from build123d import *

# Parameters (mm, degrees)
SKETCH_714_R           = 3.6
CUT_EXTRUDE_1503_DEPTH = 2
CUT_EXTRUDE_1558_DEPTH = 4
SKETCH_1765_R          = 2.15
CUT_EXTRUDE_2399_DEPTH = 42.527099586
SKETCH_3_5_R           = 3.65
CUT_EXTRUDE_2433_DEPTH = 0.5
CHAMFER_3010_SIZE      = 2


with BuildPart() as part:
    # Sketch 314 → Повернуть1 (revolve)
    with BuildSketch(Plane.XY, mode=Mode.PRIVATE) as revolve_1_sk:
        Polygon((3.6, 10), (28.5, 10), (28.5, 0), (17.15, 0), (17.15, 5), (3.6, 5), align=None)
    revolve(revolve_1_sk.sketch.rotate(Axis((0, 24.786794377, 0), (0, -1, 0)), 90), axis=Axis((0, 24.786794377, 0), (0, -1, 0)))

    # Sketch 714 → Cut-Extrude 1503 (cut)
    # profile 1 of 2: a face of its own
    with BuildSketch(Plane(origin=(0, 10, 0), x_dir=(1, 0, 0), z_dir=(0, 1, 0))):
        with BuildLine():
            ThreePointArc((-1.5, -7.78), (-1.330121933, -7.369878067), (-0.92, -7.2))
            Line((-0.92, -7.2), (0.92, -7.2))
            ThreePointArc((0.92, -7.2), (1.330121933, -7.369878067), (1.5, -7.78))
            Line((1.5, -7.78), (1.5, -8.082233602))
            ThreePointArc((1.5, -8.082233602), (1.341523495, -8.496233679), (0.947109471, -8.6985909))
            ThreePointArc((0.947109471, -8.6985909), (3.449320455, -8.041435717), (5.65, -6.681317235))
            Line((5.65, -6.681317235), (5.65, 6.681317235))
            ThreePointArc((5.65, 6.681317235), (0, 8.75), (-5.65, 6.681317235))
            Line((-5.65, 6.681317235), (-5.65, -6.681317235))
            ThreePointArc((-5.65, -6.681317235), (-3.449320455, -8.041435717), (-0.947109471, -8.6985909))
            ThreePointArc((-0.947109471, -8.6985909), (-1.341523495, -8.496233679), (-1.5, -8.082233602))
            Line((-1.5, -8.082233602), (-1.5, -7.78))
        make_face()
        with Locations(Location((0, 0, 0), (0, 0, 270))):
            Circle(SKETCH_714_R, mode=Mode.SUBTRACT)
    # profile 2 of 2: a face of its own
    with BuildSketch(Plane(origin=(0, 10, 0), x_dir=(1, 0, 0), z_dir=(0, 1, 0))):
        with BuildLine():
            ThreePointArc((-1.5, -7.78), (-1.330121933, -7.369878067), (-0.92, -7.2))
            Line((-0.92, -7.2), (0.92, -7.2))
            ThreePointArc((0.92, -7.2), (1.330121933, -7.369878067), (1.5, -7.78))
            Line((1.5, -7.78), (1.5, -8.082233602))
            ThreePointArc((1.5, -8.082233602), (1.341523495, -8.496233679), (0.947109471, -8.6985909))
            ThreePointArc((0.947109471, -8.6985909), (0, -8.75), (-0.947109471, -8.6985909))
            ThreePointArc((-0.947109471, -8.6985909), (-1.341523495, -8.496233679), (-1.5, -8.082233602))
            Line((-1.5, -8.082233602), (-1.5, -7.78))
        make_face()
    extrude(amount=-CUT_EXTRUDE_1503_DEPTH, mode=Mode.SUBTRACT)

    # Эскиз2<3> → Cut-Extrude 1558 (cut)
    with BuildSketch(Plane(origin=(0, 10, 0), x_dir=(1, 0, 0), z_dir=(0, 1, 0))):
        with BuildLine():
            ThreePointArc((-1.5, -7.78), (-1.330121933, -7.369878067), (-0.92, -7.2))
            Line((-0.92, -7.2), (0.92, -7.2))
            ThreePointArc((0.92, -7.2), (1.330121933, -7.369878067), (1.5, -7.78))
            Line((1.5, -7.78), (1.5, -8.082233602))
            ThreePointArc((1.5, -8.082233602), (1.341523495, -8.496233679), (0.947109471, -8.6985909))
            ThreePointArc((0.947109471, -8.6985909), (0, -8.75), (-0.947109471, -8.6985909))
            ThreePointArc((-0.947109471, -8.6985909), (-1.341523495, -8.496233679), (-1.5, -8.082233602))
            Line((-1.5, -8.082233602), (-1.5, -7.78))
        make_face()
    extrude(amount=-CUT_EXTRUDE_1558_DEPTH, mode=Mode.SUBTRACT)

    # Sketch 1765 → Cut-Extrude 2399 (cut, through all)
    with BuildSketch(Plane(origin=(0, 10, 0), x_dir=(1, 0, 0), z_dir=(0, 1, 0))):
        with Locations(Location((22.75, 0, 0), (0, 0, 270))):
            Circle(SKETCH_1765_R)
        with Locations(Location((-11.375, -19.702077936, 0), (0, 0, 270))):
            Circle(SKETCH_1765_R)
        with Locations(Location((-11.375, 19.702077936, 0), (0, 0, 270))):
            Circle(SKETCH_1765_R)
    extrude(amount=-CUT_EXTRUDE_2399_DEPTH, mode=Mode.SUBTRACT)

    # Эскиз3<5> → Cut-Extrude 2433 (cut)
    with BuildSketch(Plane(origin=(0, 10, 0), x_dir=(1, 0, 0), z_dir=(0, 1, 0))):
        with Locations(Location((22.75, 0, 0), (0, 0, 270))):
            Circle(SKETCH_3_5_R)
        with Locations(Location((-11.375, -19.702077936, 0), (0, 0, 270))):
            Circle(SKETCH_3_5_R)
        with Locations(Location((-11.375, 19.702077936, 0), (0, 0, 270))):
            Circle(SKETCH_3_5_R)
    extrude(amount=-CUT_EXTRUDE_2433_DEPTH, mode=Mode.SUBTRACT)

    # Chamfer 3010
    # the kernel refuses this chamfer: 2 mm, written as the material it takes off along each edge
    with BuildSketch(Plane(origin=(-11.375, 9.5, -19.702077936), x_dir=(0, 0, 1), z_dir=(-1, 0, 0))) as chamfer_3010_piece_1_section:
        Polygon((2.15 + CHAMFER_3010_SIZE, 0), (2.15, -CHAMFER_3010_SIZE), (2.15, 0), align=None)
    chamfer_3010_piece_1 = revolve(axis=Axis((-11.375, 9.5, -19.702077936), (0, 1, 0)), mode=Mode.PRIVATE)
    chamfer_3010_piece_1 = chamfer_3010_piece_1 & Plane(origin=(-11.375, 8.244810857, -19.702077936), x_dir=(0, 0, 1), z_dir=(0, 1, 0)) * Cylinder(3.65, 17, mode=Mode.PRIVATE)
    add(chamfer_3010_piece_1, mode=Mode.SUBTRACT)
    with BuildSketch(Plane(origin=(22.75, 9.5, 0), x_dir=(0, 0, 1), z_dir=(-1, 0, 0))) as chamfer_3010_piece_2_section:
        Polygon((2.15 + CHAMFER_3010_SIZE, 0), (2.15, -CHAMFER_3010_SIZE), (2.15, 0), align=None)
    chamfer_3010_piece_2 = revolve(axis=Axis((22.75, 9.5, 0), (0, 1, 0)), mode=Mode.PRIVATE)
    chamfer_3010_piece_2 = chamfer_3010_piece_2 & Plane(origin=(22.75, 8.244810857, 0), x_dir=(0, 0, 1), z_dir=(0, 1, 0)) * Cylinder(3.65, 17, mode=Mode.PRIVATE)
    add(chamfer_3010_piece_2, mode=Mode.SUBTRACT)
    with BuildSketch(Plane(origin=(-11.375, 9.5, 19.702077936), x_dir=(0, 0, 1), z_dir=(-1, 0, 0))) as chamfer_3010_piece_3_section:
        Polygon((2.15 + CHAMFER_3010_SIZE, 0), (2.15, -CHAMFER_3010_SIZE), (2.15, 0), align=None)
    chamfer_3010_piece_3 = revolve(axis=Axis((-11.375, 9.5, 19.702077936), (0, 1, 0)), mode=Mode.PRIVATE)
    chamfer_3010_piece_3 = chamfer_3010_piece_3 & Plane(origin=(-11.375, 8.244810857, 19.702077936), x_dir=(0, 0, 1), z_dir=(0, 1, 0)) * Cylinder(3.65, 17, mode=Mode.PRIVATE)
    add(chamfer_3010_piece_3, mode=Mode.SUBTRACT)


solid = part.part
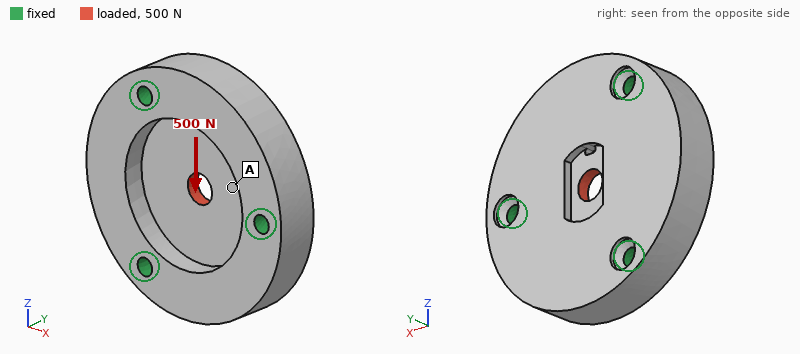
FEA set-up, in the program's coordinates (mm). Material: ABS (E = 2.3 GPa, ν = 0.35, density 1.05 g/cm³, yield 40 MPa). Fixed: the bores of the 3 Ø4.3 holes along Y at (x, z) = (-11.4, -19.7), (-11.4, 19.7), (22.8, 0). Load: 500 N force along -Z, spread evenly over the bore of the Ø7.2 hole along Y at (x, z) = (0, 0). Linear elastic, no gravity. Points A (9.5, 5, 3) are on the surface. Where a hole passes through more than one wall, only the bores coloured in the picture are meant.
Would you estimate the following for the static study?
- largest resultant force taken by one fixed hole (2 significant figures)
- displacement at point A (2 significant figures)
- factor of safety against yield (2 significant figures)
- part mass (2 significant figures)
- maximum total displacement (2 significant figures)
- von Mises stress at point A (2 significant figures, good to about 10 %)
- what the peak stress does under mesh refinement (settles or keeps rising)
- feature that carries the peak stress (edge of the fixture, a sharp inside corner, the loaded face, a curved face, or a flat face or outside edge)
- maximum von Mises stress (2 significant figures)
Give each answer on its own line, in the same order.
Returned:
170 N
18 µm
2.1
21 g
42 µm
1.3 MPa
settles
a curved face
19 MPa
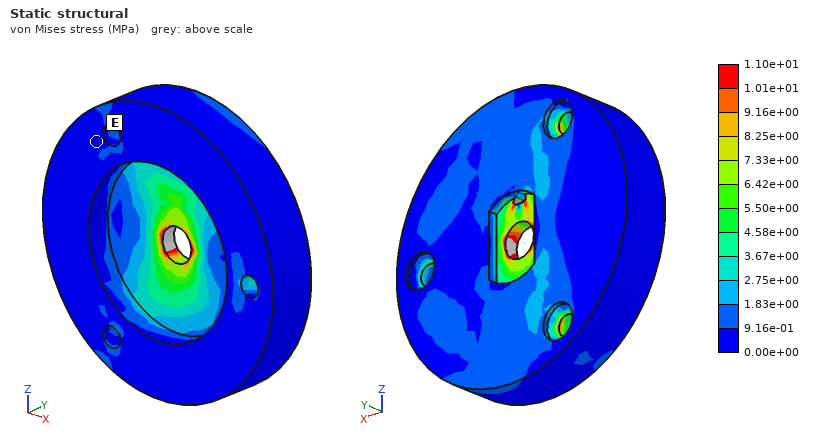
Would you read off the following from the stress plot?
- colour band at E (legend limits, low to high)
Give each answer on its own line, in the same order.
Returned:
0.00e+00 to 9.16e-01 MPa
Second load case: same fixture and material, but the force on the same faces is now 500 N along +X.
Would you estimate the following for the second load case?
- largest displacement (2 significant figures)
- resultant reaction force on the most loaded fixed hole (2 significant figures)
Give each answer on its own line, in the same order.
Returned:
42 µm
170 N
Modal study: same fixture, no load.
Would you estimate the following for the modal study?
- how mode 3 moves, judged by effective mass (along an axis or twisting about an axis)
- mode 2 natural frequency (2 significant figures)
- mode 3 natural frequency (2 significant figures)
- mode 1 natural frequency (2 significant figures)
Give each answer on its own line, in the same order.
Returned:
along Y
4200 Hz
4800 Hz
4200 Hz
